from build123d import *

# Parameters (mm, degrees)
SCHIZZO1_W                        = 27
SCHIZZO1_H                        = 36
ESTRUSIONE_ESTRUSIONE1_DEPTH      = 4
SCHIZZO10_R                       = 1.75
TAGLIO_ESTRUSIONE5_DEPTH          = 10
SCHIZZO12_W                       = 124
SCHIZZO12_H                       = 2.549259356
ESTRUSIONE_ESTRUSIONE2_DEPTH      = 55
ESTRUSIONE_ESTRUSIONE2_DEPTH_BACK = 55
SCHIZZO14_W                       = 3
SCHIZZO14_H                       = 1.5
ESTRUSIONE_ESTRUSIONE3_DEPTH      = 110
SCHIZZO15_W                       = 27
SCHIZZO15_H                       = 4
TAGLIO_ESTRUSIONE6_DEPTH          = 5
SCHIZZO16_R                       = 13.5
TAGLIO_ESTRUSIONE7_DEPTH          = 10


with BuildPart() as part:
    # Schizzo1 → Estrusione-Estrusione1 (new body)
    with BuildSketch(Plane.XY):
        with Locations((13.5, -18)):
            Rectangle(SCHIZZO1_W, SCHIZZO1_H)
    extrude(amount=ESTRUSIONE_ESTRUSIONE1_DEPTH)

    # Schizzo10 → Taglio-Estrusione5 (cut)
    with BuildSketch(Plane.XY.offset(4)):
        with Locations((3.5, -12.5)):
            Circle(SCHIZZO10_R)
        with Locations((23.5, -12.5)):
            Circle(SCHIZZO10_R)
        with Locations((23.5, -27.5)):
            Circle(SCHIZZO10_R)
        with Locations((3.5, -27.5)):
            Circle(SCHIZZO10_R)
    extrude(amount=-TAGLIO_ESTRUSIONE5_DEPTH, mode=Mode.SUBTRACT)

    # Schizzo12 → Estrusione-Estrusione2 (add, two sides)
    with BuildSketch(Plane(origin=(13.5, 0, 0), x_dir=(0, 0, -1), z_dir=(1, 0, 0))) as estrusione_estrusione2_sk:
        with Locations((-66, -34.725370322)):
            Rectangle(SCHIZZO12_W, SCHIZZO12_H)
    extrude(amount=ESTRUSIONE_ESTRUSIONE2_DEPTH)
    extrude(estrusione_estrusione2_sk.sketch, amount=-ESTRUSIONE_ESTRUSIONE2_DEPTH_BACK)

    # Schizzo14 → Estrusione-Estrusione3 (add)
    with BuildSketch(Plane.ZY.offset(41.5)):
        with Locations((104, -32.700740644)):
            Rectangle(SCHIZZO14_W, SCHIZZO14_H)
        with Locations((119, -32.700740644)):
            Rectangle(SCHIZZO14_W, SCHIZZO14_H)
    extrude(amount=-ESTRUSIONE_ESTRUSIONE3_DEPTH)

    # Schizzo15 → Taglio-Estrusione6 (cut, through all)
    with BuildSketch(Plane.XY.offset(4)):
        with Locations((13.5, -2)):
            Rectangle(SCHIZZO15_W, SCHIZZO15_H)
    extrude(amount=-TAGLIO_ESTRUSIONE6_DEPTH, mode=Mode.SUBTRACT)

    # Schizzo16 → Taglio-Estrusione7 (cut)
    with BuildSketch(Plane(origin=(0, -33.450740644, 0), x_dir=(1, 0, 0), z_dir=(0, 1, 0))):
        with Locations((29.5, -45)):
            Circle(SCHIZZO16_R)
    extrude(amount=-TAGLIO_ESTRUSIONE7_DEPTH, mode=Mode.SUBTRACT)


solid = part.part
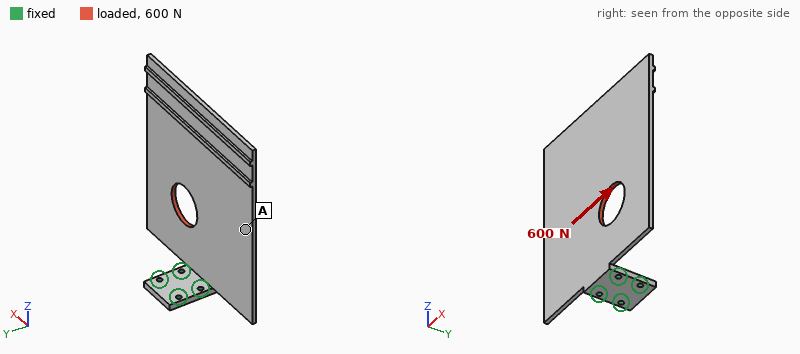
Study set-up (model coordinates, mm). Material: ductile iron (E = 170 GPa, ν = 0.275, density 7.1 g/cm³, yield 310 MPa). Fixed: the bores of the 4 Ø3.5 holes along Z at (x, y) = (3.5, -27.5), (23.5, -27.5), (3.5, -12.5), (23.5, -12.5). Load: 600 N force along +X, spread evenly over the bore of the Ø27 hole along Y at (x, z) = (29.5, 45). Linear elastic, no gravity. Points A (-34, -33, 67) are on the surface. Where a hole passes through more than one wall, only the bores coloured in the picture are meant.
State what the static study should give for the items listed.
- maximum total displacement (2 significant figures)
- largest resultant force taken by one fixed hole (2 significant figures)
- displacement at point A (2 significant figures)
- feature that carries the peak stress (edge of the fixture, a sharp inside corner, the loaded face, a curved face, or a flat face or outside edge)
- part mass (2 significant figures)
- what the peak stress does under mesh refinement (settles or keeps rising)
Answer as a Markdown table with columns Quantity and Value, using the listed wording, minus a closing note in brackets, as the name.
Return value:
| Quantity | Value |
|---|---|
| maximum total displacement | 0.23 mm |
| largest resultant force taken by one fixed hole | 1.3 kN |
| displacement at point A | 0.14 mm |
| feature that carries the peak stress | edge of the fixture |
| part mass | 270 g |
| what the peak stress does under mesh refinement | keeps rising |
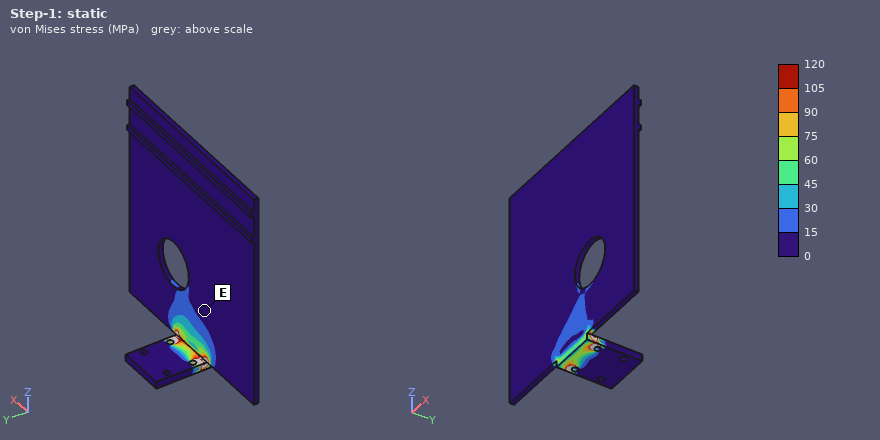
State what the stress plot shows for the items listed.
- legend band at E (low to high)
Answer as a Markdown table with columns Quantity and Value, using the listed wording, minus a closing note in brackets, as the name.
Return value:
| Quantity | Value |
|---|---|
| legend band at E | 0 to 15 MPa |
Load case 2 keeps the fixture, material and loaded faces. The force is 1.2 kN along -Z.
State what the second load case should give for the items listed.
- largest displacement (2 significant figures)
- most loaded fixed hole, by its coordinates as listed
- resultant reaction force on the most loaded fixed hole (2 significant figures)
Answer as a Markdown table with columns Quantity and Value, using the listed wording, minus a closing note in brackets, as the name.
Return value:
| Quantity | Value |
|---|---|
| largest displacement | 0.28 mm |
| most loaded fixed hole, by its coordinates as listed | (23.5, -27.5) |
| resultant reaction force on the most loaded fixed hole | 1.6 kN |
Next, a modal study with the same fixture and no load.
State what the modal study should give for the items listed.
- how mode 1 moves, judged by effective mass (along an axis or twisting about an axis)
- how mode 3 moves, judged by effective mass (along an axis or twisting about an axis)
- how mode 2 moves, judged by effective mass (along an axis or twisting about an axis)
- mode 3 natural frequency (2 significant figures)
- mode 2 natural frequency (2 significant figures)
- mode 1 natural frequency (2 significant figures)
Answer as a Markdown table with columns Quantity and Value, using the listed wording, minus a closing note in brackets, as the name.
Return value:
| Quantity | Value |
|---|---|
| how mode 1 moves, judged by effective mass | along Y |
| how mode 3 moves, judged by effective mass | along X |
| how mode 2 moves, judged by effective mass | twisting about Z |
| mode 3 natural frequency | 510 Hz |
| mode 2 natural frequency | 220 Hz |
| mode 1 natural frequency | 87 Hz |
